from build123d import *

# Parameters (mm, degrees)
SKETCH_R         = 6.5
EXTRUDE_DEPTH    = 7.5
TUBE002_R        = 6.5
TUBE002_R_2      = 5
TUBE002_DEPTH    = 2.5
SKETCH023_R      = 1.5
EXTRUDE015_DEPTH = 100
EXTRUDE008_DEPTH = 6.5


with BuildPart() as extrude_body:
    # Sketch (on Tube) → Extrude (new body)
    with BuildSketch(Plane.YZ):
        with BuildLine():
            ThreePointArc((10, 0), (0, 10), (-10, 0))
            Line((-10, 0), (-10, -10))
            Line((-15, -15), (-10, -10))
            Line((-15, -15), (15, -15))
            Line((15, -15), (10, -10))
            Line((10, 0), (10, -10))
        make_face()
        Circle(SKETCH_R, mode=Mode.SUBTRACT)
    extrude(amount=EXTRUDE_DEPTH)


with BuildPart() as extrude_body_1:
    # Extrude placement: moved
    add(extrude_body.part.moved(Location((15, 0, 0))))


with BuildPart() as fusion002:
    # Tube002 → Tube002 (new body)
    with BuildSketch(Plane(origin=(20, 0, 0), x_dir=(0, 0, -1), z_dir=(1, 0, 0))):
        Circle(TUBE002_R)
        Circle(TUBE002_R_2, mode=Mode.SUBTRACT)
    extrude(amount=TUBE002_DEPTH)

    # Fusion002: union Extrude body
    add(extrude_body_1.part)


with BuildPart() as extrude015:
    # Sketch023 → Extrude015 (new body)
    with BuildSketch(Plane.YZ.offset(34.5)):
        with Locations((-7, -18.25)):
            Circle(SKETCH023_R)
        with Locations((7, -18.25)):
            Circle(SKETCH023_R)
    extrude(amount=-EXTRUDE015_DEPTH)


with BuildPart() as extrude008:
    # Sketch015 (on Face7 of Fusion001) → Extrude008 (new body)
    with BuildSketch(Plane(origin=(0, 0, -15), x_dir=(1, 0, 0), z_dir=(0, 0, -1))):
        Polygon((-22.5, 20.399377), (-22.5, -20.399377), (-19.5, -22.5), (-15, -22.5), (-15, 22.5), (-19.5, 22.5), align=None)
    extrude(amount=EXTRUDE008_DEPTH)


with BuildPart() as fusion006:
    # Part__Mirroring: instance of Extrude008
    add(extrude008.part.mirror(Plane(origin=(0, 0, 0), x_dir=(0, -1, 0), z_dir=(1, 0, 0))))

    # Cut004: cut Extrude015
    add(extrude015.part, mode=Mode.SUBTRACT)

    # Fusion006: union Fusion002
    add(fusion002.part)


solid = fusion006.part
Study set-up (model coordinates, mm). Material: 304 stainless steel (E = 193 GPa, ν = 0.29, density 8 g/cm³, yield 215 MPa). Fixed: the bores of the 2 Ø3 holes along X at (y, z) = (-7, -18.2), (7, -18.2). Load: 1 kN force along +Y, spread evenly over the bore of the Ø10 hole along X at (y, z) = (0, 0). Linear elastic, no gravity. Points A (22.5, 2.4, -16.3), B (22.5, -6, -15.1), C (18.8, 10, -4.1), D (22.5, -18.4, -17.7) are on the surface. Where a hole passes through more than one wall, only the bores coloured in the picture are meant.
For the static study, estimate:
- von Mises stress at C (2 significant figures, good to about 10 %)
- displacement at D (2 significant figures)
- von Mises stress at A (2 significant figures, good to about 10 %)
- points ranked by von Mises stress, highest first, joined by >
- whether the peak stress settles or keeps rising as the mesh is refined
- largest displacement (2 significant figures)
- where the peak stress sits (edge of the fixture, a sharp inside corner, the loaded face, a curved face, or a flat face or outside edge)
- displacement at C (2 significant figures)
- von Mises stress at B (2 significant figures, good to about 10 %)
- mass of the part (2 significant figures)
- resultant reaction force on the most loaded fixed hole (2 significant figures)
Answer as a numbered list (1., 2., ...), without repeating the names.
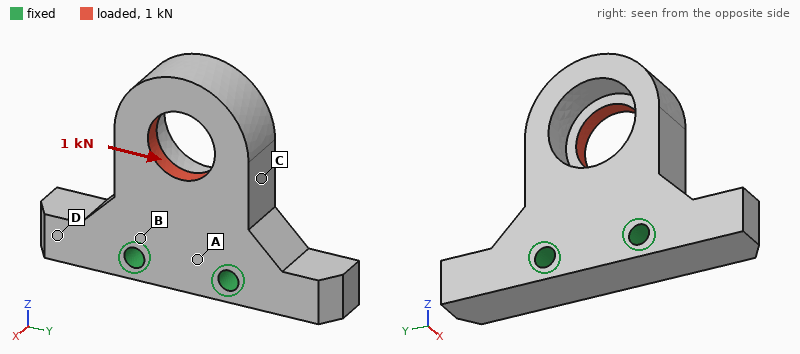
1. 35 MPa
2. 1.6 µm
3. 15 MPa
4. C > B > A > D
5. keeps rising
6. 10 µm
7. edge of the fixture
8. 4.0 µm
9. 21 MPa
10. 38 g
11. 1.2 kN
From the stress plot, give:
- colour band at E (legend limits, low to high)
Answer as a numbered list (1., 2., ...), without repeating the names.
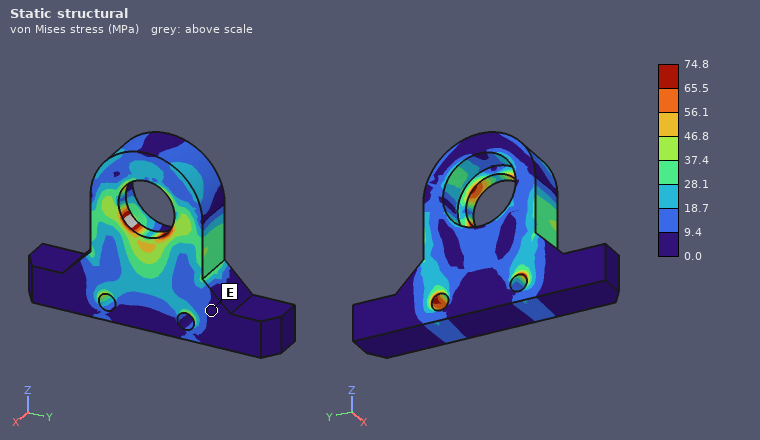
1. 0.0 to 9.4 MPa
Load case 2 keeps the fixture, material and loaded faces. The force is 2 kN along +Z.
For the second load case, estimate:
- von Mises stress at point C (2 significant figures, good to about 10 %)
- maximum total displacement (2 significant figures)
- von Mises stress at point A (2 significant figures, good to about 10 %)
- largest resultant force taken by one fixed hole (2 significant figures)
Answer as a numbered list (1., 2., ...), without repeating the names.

1. 15 MPa
2. 16 µm
3. 19 MPa
4. 1.0 kN
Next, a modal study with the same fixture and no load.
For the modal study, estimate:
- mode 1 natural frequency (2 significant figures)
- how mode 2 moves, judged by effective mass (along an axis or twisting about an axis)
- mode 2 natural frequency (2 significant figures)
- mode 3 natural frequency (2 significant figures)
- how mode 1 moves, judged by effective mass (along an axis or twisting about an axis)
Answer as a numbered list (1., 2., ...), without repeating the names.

1. 9100 Hz
2. along Y
3. 16 kHz
4. 21 kHz
5. along X
